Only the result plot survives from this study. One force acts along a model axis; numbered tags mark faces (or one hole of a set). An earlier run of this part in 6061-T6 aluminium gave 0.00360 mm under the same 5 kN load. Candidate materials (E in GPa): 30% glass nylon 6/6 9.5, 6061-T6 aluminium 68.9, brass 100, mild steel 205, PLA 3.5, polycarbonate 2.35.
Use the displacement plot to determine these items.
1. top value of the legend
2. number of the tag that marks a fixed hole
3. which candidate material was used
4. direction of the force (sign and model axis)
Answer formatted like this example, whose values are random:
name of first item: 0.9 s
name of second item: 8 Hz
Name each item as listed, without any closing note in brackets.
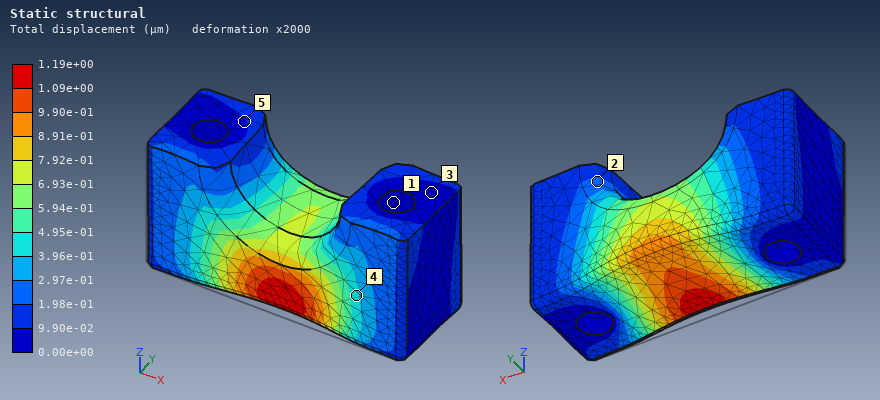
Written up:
top value of the legend: 1.19e+00 µm
number of the tag that marks a fixed hole: 1
which candidate material was used: mild steel
direction of the force: +Y
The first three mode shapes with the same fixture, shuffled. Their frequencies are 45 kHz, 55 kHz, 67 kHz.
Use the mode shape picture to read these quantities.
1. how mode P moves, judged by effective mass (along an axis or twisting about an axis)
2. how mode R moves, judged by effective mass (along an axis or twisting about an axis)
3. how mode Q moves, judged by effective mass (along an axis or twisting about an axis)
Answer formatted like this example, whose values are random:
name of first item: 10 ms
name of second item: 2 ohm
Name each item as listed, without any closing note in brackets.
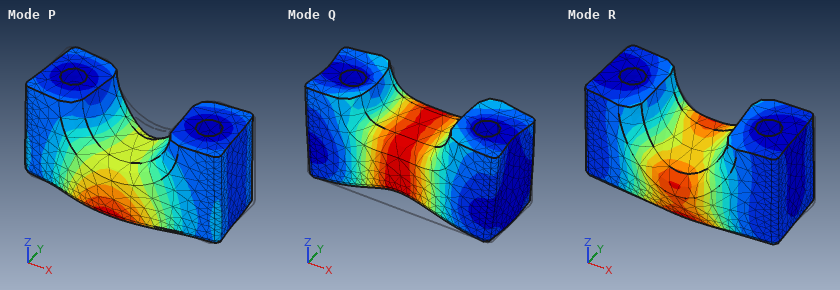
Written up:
how mode P moves, judged by effective mass: along Y
how mode R moves, judged by effective mass: twisting about X
how mode Q moves, judged by effective mass: along Z
